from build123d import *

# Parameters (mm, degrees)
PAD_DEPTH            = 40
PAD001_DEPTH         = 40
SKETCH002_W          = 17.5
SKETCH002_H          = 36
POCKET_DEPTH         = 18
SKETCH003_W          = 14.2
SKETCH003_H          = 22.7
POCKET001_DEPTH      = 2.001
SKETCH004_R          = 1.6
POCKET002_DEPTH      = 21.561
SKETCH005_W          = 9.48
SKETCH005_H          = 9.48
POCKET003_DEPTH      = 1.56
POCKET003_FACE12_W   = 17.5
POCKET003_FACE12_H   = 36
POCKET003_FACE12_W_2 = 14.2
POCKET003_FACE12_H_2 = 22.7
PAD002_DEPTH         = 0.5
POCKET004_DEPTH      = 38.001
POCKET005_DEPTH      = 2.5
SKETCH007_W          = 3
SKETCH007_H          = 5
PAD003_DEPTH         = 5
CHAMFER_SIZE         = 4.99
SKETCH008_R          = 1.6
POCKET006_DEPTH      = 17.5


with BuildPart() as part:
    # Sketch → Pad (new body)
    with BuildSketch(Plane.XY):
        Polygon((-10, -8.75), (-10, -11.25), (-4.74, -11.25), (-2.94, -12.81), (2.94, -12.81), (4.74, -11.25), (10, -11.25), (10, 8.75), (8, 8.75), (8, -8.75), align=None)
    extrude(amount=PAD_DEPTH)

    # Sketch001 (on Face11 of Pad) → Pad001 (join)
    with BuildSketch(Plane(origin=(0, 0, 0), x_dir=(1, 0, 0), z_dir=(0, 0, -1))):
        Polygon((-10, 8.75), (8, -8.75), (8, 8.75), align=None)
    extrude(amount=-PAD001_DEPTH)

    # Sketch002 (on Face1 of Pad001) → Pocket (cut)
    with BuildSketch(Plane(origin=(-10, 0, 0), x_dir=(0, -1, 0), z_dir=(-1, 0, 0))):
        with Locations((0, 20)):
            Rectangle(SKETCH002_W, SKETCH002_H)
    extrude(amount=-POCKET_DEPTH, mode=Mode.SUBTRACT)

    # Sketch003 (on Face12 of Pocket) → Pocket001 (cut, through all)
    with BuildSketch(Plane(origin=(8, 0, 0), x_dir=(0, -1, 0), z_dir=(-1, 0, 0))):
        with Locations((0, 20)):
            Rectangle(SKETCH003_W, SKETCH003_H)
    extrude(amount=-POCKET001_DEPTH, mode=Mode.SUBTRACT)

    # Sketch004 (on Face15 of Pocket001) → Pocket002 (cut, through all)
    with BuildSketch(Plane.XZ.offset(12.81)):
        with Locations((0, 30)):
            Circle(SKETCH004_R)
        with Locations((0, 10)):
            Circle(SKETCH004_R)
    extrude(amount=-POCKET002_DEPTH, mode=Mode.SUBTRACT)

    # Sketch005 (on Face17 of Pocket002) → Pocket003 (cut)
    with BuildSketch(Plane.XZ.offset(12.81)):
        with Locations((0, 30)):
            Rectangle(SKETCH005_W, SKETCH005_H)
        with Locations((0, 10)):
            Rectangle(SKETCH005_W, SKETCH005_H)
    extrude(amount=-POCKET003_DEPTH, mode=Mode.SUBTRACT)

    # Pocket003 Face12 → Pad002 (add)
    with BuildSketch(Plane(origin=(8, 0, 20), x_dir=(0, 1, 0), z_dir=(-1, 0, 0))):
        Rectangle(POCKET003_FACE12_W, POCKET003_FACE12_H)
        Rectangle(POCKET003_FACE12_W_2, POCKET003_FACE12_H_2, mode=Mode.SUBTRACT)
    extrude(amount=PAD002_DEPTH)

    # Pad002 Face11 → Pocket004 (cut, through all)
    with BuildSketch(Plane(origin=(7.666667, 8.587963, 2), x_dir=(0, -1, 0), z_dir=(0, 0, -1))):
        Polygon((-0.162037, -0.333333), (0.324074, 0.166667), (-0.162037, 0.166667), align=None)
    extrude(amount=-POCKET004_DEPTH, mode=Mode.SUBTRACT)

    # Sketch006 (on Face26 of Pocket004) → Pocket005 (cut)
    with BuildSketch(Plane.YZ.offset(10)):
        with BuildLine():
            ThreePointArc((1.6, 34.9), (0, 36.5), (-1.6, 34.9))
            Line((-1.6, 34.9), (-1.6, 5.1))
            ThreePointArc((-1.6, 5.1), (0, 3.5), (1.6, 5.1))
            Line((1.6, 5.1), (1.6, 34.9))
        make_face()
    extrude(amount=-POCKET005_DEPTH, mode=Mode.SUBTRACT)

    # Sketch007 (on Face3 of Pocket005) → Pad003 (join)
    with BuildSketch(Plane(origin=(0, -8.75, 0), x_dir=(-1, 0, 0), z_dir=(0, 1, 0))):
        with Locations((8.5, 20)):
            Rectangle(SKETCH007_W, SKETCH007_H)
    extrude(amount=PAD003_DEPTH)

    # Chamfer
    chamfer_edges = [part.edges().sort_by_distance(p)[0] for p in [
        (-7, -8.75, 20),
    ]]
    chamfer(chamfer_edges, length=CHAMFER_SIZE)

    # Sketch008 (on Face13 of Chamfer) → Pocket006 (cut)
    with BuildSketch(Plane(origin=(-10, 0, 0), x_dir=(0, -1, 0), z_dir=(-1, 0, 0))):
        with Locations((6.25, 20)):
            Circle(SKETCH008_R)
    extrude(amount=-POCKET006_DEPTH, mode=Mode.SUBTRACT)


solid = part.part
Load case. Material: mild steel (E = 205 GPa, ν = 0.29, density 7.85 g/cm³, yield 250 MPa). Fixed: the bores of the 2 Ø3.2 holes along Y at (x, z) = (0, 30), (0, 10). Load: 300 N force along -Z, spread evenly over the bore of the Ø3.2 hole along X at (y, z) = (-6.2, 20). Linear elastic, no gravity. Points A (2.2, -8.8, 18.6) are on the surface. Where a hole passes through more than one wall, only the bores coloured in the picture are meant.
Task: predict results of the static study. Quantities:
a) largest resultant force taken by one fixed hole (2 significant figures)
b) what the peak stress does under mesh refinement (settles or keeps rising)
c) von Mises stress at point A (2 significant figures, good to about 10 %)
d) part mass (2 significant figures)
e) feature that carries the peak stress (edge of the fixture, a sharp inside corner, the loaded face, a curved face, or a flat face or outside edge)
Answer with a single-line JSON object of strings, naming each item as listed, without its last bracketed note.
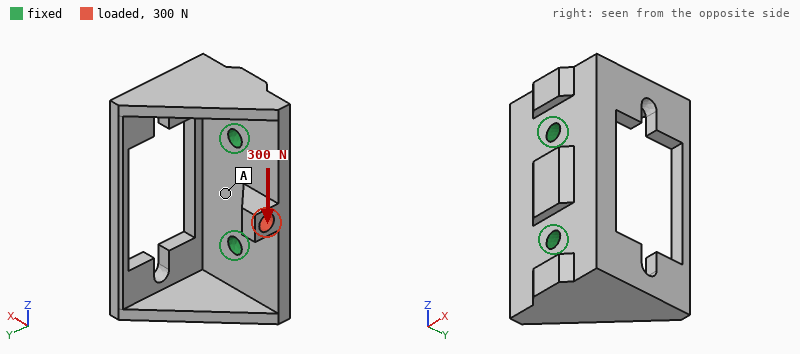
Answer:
{"largest resultant force taken by one fixed hole": "190 N", "what the peak stress does under mesh refinement": "keeps rising", "von Mises stress at point A": "6.8 MPa", "part mass": "30 g", "feature that carries the peak stress": "a sharp inside corner"}
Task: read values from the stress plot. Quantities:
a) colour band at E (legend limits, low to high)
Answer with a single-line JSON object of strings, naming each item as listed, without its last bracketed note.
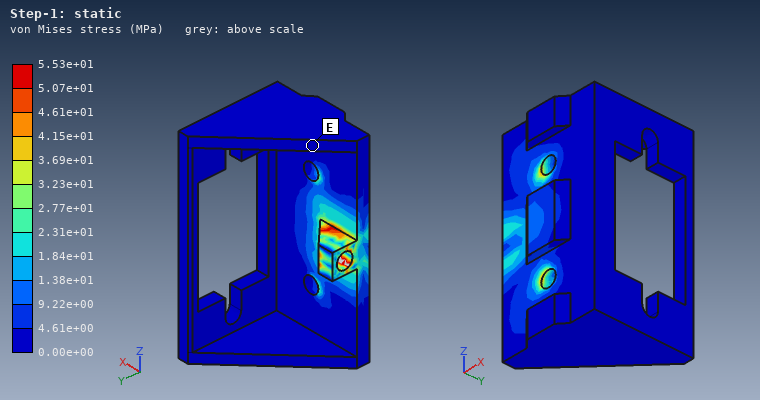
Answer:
{"colour band at E": "0.00e+00 to 4.61e+00 MPa"}
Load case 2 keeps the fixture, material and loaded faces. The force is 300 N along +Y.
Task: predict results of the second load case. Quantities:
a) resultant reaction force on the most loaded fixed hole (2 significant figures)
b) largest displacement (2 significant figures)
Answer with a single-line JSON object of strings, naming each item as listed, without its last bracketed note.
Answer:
{"resultant reaction force on the most loaded fixed hole": "160 N", "largest displacement": "13 µm"}
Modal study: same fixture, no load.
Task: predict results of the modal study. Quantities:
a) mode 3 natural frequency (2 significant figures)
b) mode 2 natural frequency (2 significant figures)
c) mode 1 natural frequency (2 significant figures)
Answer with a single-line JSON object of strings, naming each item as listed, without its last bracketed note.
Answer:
{"mode 3 natural frequency": "8300 Hz", "mode 2 natural frequency": "5500 Hz", "mode 1 natural frequency": "5400 Hz"}
